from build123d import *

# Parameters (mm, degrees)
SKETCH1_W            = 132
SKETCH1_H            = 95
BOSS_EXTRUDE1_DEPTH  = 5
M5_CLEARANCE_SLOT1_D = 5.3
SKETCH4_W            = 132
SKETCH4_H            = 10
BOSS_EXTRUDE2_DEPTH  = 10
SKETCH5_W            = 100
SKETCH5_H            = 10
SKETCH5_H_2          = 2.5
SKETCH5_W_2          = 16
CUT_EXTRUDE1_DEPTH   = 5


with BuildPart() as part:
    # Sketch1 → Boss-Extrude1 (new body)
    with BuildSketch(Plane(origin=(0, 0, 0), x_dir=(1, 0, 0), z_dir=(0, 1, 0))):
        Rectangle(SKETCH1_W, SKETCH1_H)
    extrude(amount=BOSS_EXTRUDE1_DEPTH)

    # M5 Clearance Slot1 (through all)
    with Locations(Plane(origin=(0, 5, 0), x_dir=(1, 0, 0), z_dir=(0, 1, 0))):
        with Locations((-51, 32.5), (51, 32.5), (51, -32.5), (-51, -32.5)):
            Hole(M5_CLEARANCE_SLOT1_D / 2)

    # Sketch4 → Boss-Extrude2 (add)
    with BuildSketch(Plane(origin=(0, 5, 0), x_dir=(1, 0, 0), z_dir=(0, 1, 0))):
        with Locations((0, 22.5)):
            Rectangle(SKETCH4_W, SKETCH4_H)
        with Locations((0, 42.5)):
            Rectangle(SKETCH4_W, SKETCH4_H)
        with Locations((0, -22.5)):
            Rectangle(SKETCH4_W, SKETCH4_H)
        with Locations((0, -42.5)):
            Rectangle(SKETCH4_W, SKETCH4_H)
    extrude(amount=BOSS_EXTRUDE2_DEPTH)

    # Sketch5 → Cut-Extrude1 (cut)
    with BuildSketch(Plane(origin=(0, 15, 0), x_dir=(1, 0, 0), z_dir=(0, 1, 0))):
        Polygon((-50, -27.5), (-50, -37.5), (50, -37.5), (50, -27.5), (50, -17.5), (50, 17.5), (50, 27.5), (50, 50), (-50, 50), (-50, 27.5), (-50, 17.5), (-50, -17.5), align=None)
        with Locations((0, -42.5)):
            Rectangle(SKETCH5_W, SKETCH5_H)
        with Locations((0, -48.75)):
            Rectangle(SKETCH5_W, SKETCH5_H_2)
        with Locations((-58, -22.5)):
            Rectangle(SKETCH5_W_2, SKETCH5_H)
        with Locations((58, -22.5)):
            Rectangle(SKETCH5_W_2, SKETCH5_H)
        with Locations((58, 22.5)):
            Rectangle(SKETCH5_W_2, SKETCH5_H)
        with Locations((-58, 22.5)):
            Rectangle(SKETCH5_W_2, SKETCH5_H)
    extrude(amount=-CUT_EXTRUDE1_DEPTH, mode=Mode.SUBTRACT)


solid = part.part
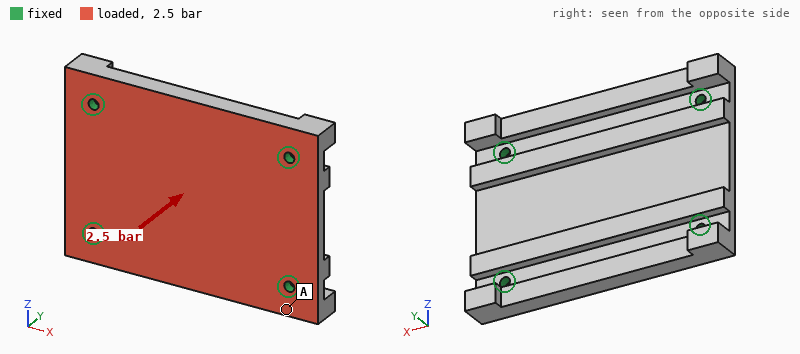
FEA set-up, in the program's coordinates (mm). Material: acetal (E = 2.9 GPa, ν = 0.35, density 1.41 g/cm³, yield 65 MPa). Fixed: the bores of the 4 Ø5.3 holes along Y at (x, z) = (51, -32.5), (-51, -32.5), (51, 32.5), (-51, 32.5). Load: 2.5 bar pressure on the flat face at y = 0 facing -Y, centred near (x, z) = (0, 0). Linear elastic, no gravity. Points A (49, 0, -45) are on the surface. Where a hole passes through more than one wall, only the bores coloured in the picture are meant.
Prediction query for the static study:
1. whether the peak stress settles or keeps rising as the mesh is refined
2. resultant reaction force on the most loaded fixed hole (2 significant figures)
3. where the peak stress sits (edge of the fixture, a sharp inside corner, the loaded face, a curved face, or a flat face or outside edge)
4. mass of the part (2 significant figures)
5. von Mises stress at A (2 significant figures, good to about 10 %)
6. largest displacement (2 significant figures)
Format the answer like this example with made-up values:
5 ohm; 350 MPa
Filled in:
keeps rising; 850 N; edge of the fixture; 130 g; 6.4 MPa; 1.5 mm
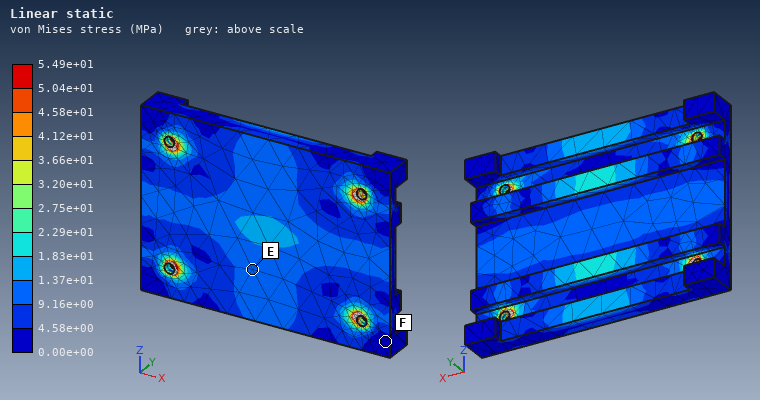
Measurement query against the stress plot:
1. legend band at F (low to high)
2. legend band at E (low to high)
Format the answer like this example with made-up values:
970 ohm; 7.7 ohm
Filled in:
0.00e+00 to 4.58e+00 MPa; 9.16e+00 to 1.37e+01 MPa
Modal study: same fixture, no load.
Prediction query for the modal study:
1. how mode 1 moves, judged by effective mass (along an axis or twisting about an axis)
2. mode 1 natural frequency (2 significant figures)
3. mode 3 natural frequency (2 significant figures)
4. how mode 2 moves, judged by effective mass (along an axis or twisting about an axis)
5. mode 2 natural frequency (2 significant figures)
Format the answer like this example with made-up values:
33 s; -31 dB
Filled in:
along Y; 830 Hz; 1300 Hz; twisting about X; 1100 Hz
